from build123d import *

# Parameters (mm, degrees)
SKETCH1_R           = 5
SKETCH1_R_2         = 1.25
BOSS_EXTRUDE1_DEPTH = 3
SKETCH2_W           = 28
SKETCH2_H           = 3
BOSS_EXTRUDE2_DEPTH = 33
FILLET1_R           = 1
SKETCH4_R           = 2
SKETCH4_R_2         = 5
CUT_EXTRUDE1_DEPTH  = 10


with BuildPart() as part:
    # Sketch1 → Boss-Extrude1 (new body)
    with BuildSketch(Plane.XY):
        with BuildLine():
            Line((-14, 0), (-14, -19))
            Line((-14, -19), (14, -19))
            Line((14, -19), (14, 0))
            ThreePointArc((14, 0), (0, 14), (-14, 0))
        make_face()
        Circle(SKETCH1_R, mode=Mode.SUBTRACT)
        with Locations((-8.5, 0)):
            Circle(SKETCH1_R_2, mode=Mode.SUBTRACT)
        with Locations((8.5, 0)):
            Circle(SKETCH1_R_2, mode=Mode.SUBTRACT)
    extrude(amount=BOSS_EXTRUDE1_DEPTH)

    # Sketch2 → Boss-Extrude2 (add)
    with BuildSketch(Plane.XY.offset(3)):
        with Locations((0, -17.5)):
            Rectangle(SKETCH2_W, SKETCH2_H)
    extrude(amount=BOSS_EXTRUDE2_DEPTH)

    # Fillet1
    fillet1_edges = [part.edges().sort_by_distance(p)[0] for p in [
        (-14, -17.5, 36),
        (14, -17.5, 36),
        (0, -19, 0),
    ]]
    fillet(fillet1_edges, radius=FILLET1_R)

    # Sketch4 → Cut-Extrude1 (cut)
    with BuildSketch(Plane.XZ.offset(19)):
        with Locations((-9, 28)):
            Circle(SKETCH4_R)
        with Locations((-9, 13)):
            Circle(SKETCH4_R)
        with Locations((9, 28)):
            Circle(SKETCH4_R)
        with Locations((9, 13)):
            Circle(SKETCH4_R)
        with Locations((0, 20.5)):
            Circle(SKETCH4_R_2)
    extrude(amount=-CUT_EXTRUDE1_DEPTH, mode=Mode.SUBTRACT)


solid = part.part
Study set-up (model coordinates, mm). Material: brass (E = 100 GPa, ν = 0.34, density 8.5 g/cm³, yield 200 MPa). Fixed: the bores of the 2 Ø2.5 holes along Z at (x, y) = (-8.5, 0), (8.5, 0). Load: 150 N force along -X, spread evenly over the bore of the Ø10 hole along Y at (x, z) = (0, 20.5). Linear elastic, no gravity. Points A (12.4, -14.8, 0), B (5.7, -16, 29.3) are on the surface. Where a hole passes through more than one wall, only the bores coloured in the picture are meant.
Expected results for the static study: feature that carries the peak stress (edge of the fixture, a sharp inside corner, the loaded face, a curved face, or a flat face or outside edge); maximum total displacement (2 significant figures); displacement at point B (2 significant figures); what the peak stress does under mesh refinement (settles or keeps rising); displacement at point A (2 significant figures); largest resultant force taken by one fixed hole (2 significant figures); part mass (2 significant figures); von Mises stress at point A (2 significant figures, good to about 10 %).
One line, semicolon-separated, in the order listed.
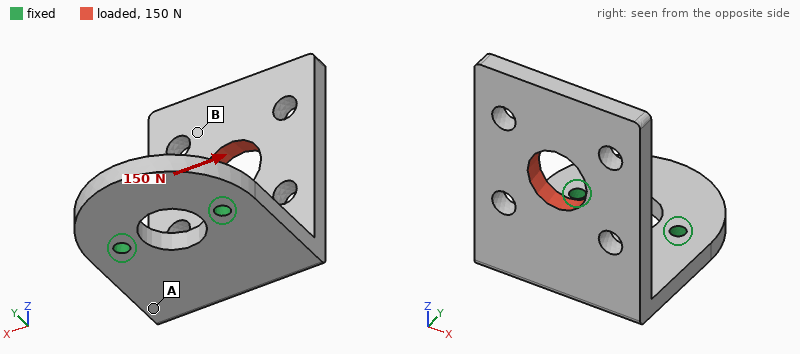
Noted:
edge of the fixture; 0.11 mm; 0.086 mm; keeps rising; 0.030 mm; 200 N; 39 g; 33 MPa
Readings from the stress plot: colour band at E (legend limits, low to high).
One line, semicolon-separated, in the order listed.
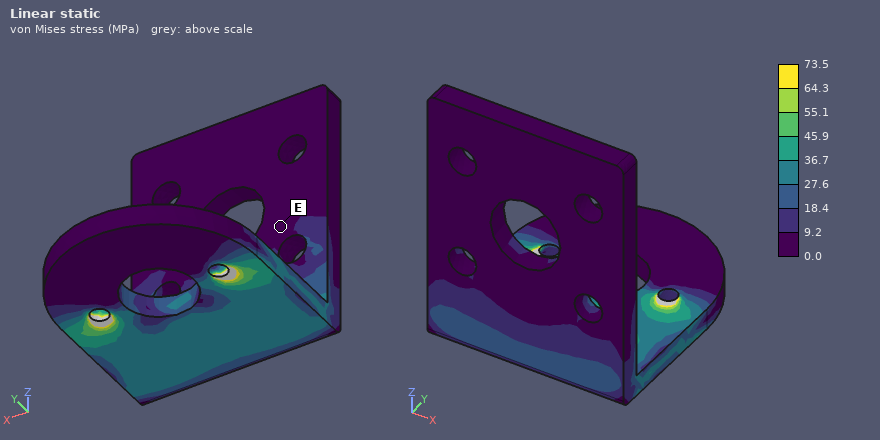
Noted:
0.0 to 9.2 MPa
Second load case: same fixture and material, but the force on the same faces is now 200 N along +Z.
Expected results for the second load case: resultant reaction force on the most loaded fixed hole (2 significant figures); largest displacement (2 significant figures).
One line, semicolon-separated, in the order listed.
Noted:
100 N; 0.22 mm
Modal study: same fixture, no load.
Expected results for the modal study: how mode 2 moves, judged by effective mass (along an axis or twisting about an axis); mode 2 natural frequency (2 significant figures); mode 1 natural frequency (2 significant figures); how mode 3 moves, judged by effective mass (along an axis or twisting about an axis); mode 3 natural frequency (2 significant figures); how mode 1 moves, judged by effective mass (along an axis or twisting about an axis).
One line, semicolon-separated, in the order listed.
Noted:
along X; 1500 Hz; 770 Hz; along Z; 2500 Hz; along Y
